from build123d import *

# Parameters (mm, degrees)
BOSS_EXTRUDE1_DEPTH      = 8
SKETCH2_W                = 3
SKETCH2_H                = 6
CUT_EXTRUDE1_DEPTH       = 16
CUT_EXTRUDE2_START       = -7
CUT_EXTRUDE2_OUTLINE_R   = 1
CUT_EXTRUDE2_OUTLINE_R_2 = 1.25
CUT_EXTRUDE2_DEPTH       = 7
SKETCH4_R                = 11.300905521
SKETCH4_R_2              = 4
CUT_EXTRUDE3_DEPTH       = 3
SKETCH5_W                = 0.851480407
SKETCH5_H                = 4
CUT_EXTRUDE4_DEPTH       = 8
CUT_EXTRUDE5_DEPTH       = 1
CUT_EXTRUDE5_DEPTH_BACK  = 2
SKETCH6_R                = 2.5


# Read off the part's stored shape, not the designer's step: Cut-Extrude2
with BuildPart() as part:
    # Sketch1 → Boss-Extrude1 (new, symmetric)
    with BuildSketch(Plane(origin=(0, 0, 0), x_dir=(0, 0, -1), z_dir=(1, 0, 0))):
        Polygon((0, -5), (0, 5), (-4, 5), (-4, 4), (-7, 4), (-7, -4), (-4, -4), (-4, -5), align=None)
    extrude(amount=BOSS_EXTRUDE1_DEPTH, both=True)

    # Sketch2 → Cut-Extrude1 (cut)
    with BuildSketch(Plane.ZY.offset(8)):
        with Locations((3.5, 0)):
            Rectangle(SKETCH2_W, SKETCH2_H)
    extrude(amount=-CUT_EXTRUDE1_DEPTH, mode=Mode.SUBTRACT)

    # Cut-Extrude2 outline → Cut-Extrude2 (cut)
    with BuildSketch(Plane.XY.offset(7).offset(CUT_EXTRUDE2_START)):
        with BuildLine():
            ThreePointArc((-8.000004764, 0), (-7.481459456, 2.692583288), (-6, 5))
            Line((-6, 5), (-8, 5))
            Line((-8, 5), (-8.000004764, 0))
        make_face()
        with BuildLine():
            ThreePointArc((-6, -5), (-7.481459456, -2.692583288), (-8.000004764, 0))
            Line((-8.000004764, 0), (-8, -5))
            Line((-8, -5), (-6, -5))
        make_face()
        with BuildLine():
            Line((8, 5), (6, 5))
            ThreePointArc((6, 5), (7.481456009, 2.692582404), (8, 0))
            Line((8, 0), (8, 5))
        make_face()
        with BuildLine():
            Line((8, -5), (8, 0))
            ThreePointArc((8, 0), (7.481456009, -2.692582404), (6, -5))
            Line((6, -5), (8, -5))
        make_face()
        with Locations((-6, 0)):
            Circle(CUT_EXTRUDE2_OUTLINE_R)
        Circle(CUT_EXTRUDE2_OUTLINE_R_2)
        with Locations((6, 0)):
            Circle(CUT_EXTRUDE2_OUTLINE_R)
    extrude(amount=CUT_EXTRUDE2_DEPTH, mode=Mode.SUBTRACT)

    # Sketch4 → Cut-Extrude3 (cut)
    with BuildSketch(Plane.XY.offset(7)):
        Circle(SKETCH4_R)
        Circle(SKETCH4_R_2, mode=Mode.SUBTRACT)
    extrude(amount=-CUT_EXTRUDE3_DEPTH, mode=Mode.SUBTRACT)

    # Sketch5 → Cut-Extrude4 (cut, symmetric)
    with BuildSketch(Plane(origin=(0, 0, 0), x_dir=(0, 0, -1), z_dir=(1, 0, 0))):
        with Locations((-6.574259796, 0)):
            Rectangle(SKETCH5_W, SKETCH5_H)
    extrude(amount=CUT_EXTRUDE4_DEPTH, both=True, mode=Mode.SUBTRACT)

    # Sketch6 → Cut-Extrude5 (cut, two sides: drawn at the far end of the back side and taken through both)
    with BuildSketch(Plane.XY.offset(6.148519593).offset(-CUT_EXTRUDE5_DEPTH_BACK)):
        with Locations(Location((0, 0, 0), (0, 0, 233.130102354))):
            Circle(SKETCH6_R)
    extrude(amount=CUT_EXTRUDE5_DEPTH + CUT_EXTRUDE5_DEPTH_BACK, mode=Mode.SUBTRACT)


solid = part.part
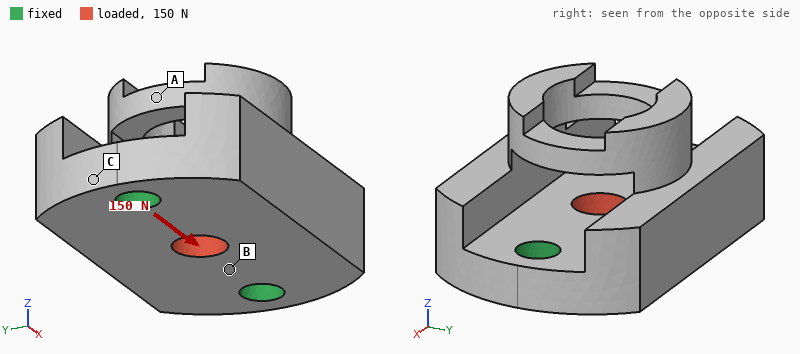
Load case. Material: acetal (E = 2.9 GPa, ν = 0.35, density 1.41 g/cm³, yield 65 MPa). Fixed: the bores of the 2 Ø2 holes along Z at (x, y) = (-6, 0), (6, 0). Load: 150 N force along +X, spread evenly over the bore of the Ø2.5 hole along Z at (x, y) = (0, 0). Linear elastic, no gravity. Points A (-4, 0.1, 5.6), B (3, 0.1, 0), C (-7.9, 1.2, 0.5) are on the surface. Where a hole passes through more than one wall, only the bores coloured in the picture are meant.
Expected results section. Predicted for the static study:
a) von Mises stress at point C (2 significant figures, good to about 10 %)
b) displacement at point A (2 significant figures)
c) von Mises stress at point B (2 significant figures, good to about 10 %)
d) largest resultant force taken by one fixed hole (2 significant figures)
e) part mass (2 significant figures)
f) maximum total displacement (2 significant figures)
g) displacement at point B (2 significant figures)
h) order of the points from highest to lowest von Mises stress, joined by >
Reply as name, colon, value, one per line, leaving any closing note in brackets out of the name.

von Mises stress at point C: 3.1 MPa
displacement at point A: 6.7 µm
von Mises stress at point B: 10 MPa
largest resultant force taken by one fixed hole: 75 N
part mass: 0.62 g
maximum total displacement: 15 µm
displacement at point B: 7.4 µm
order of the points from highest to lowest von Mises stress, joined by >: B > C > A
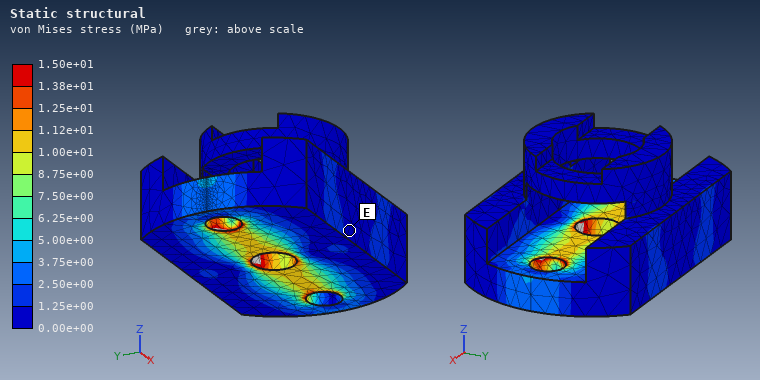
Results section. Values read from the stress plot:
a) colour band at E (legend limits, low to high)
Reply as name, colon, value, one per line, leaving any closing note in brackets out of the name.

colour band at E: 0.00e+00 to 1.25e+00 MPa
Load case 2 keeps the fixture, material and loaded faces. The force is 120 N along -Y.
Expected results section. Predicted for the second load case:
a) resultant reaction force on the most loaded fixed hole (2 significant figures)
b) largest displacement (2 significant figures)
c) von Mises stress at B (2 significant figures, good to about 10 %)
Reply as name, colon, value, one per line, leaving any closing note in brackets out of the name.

resultant reaction force on the most loaded fixed hole: 60 N
largest displacement: 24 µm
von Mises stress at B: 4.5 MPa
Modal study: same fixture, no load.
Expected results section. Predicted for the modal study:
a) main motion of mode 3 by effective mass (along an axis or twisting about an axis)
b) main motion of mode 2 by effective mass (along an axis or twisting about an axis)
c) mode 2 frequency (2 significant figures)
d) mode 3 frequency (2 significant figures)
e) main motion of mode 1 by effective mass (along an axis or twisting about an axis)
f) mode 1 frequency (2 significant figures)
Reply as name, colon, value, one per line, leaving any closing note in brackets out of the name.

main motion of mode 3 by effective mass: along X
main motion of mode 2 by effective mass: along Z
mode 2 frequency: 11 kHz
mode 3 frequency: 15 kHz
main motion of mode 1 by effective mass: along Y
mode 1 frequency: 7600 Hz
